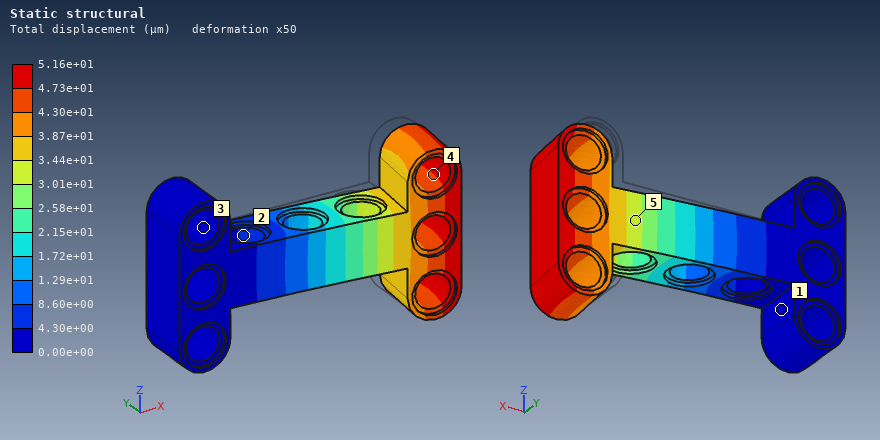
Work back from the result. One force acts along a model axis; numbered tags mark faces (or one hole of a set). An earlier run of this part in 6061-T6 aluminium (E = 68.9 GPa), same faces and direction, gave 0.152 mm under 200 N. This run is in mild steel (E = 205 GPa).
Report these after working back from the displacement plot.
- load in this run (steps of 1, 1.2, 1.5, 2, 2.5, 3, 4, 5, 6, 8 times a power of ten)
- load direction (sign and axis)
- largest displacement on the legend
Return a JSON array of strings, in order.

["200 N", "-Y", "5.16e+01 µm"]
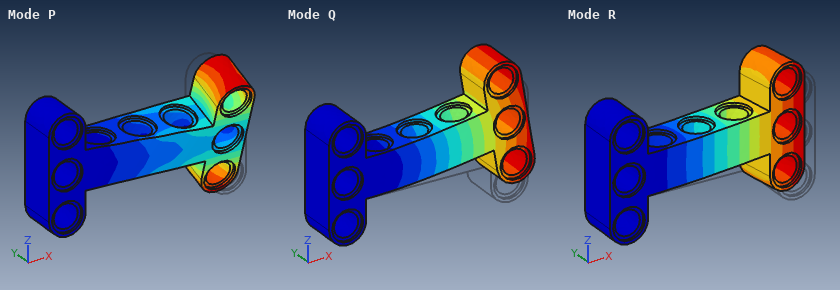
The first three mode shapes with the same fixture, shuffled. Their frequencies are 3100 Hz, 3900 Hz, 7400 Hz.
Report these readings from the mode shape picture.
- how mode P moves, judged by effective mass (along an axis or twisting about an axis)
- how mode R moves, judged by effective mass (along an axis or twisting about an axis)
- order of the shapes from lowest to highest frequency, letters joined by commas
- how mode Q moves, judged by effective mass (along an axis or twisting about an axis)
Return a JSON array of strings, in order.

["twisting about X", "along Y", "Q, R, P", "along Z"]
